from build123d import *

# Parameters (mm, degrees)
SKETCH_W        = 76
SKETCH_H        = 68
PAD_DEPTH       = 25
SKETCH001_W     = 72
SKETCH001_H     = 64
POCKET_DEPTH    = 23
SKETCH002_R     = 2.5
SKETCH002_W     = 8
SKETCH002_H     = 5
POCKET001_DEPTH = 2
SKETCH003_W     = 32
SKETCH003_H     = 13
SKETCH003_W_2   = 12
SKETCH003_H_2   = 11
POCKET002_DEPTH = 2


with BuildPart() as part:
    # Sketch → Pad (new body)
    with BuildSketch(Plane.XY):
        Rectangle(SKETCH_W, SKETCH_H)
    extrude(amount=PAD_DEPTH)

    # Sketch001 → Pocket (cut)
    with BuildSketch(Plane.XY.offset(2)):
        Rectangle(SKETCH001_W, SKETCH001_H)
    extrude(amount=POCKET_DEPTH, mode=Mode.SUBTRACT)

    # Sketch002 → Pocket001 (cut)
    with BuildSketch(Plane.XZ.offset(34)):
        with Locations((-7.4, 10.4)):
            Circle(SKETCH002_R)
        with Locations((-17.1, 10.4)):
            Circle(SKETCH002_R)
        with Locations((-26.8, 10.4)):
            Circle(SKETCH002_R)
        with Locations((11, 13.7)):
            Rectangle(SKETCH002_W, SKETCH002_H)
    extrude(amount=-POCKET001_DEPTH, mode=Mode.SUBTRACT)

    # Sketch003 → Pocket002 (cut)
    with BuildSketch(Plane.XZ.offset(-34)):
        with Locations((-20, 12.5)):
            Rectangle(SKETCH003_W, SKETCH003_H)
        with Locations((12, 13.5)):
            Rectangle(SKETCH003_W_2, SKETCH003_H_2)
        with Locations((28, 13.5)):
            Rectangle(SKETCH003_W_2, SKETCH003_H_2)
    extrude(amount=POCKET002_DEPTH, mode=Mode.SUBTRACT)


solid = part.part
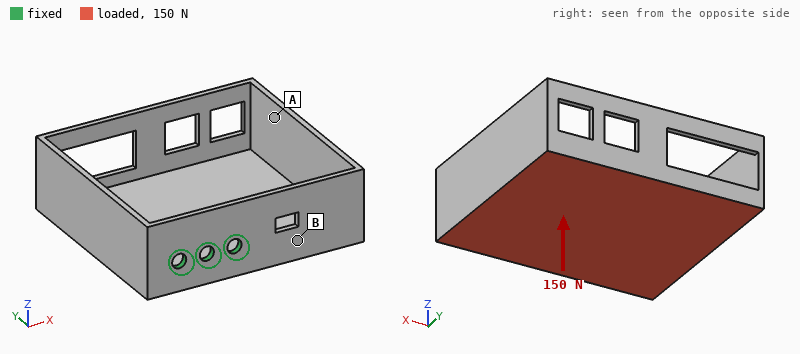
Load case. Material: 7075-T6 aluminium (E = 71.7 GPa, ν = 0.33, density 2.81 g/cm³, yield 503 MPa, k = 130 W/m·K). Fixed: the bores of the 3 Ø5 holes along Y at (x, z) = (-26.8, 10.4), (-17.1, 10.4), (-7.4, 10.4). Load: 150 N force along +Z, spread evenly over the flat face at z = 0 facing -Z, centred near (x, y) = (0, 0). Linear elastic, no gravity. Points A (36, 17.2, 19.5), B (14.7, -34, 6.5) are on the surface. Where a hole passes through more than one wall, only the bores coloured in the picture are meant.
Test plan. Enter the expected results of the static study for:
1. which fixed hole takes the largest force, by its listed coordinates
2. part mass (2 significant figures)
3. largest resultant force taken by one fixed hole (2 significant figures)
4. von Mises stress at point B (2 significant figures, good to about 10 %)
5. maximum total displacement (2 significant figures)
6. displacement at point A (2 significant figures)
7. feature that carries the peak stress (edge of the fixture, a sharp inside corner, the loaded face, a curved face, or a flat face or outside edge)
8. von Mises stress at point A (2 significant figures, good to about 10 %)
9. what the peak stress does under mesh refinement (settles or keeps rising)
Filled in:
(-7.4, 10.4)
61 g
190 N
33 MPa
1.1 mm
0.85 mm
edge of the fixture
14 MPa
keeps rising
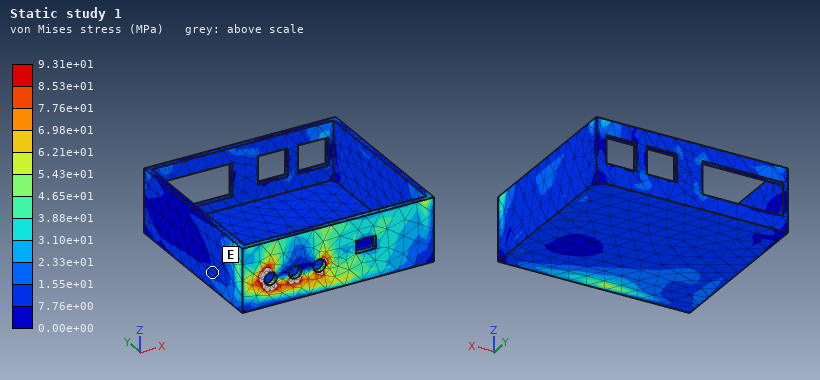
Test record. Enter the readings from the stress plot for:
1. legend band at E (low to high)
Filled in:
7.76e+00 to 1.55e+01 MPa
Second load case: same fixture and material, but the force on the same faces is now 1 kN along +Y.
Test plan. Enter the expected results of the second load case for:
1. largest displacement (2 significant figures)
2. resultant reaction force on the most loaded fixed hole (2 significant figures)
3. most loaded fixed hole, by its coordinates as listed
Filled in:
1.1 mm
980 N
(-7.4, 10.4)
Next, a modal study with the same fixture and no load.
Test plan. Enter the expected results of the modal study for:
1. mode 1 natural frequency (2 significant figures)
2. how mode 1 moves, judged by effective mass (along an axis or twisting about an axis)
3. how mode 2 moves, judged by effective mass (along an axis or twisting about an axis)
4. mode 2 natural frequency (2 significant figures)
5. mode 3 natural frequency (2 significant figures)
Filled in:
310 Hz
along Z
along X
560 Hz
960 Hz
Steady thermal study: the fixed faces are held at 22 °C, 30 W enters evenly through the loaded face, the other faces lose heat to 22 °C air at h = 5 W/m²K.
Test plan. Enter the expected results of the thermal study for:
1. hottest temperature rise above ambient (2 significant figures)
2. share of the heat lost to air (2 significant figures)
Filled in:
56 K
11 %
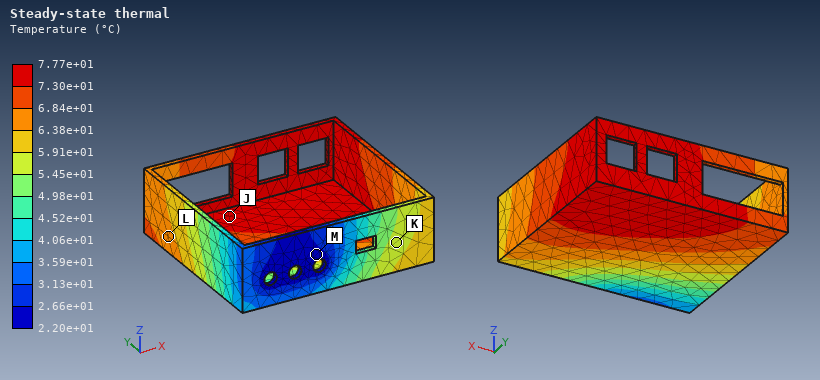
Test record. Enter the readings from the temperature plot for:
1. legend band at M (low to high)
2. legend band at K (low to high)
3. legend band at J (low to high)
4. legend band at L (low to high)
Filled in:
2.20e+01 to 2.66e+01 °C
5.45e+01 to 5.91e+01 °C
7.30e+01 to 7.77e+01 °C
6.38e+01 to 6.84e+01 °C
